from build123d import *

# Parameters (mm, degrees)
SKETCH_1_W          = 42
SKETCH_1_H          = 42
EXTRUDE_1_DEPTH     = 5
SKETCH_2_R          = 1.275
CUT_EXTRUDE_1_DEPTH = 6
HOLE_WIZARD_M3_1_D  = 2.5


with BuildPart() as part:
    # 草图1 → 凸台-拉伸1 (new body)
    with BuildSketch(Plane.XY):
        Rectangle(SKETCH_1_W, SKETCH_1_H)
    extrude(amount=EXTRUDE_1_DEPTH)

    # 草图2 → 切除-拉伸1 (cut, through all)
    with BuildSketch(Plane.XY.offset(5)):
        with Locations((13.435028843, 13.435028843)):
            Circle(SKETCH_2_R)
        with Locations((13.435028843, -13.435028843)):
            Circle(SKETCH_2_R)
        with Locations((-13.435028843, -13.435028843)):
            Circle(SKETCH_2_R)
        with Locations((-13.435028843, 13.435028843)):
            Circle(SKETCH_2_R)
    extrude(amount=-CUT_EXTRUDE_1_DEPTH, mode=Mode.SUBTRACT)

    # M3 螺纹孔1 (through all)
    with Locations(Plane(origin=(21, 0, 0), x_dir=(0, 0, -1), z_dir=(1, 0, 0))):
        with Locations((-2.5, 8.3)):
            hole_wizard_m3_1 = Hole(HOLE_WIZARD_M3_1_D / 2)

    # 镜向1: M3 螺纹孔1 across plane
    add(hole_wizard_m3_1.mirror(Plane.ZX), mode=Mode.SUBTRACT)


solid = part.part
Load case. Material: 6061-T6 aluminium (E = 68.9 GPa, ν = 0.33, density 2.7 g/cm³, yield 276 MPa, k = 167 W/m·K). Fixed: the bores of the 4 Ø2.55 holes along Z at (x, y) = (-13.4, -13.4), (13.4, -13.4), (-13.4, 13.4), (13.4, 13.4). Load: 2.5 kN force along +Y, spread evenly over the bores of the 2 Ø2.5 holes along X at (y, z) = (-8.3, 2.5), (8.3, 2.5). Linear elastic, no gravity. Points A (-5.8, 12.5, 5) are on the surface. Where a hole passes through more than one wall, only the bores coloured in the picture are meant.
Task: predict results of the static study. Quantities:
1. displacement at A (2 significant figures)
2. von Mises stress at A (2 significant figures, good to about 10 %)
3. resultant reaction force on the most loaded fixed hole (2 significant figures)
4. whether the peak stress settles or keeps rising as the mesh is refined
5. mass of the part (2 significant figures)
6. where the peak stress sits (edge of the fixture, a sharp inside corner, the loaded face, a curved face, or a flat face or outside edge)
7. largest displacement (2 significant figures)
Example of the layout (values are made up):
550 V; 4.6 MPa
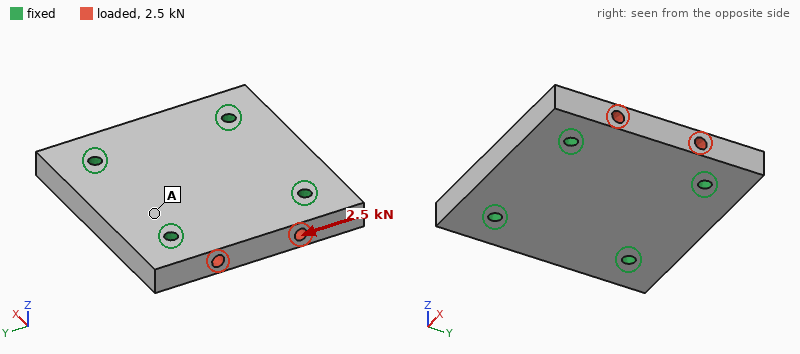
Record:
1.6 µm; 4.0 MPa; 630 N; keeps rising; 22 g; edge of the fixture; 2.0 µm
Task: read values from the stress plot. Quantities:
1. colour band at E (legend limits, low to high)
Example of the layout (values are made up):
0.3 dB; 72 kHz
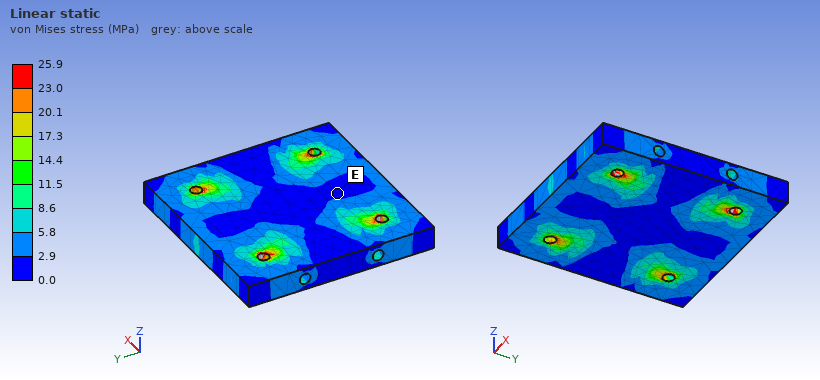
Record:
0.0 to 2.9 MPa
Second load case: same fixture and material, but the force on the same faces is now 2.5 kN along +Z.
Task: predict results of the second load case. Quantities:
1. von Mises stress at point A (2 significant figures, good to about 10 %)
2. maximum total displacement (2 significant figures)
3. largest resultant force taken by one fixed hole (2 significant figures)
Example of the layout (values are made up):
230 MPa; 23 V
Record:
8.5 MPa; 12 µm; 630 N
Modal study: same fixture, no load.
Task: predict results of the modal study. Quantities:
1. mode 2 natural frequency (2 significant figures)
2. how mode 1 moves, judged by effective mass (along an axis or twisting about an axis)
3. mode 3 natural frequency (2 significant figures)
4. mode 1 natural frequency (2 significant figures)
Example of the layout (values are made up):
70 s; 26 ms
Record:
26 kHz; along Z; 26 kHz; 20 kHz
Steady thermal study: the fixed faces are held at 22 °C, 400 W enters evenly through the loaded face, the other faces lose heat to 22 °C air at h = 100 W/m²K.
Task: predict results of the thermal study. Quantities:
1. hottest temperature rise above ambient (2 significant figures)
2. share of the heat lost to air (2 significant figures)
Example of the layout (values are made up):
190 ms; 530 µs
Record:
65 K; 3.9 %
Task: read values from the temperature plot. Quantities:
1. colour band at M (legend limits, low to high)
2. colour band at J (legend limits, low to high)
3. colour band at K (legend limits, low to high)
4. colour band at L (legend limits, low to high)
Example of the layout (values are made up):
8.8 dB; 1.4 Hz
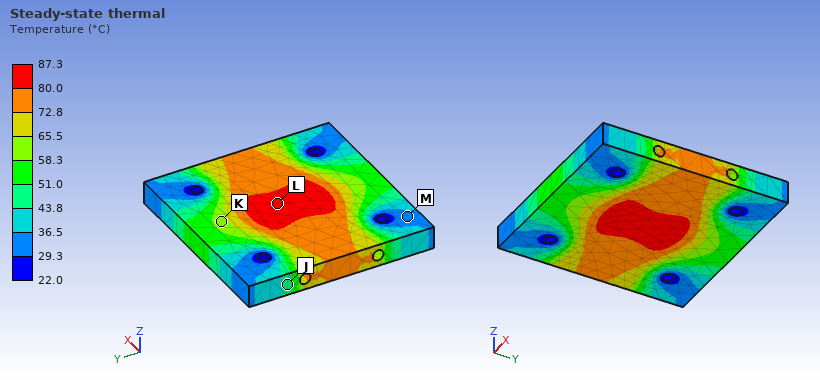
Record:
29.3 to 36.5 °C; 43.8 to 51.0 °C; 58.3 to 65.5 °C; 80.0 to 87.3 °C
